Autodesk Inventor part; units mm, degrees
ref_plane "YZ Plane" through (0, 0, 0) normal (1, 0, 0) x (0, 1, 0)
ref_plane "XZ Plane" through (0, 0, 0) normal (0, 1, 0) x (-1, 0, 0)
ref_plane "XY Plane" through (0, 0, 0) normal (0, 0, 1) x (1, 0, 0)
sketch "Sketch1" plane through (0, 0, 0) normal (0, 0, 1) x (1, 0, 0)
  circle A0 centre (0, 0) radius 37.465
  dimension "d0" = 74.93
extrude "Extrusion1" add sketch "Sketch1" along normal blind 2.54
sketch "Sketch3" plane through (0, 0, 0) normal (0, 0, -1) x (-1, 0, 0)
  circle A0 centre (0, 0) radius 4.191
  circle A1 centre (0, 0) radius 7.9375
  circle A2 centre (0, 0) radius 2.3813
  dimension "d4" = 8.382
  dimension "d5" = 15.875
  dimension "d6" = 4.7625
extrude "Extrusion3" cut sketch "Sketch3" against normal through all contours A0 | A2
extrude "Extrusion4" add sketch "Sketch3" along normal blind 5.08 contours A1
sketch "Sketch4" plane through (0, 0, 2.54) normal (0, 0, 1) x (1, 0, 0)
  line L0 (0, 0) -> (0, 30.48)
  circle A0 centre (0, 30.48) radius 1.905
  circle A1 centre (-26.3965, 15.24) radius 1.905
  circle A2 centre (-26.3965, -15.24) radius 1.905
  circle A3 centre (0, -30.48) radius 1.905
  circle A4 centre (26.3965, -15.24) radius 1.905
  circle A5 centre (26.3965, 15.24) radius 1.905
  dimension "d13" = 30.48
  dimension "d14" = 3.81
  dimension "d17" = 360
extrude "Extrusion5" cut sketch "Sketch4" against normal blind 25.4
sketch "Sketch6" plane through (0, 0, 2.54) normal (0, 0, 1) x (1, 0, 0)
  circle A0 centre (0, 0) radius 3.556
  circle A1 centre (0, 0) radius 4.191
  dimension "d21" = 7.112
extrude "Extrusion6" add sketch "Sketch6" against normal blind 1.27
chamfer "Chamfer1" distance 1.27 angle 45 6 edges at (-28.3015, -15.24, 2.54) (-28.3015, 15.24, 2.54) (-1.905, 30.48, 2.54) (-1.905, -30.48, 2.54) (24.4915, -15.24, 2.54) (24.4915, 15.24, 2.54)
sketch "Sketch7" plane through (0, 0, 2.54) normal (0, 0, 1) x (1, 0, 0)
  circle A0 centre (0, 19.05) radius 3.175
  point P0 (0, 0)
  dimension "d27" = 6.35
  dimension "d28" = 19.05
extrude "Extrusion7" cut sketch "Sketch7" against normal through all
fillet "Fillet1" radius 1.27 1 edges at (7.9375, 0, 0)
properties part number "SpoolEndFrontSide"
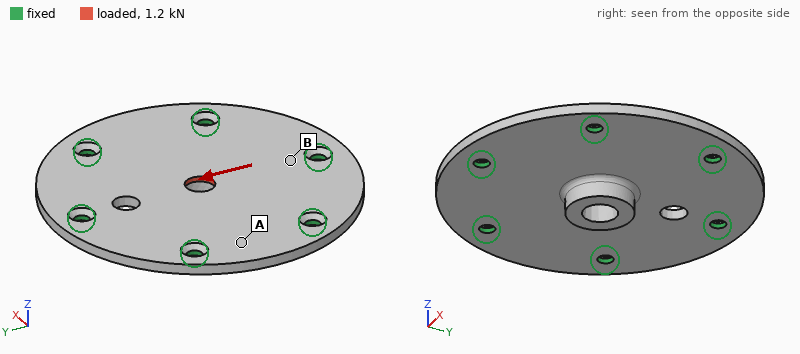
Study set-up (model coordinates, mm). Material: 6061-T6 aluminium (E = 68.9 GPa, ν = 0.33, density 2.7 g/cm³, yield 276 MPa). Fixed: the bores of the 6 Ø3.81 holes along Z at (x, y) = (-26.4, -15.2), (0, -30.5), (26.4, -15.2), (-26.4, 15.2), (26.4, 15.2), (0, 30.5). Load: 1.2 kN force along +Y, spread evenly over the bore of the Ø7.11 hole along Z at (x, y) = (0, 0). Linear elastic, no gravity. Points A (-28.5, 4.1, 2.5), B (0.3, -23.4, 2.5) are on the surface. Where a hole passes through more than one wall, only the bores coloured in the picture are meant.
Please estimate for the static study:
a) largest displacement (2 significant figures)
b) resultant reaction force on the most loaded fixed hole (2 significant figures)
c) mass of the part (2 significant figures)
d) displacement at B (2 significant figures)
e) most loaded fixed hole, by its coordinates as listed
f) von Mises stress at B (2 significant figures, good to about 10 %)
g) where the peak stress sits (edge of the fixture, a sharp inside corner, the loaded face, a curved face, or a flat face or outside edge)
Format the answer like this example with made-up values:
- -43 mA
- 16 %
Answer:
- 6.4 µm
- 310 N
- 31 g
- 1.1 µm
- (0, -30.5)
- 9.6 MPa
- the loaded face
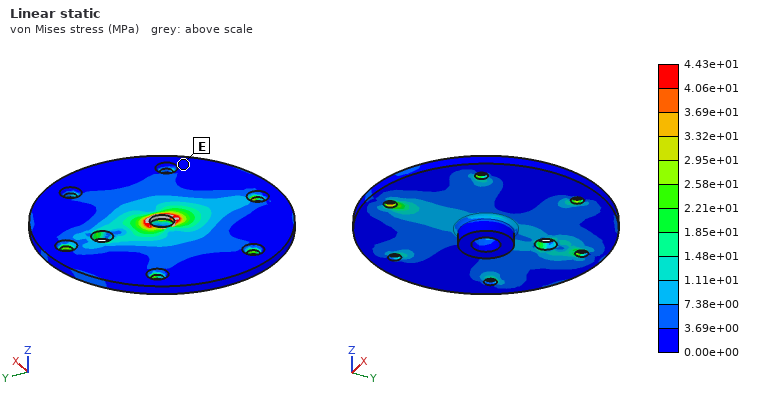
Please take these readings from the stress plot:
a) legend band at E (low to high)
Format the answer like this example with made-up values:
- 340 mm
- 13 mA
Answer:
- 0.00e+00 to 3.69e+00 MPa
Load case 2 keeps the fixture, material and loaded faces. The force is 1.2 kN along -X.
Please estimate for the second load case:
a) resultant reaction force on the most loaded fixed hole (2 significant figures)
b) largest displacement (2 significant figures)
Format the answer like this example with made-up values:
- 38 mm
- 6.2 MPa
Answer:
- 270 N
- 6.0 µm
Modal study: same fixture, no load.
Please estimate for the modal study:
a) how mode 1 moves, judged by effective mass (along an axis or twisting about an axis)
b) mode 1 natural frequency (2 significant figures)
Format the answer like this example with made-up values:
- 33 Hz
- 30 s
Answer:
- along Z
- 5200 Hz
